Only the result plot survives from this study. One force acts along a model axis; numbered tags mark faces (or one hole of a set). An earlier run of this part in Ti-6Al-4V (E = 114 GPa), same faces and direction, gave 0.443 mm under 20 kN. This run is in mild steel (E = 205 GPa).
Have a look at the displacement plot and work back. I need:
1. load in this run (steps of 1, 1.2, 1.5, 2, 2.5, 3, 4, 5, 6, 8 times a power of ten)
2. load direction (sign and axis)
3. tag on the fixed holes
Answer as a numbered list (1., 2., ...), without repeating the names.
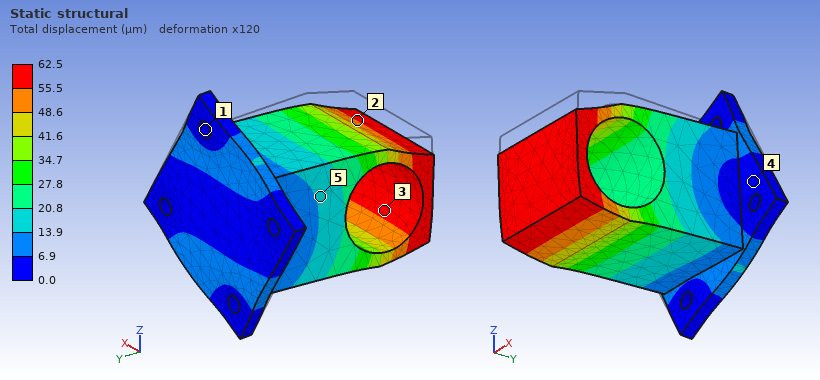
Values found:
1. 5 kN
2. -Z
3. 1
